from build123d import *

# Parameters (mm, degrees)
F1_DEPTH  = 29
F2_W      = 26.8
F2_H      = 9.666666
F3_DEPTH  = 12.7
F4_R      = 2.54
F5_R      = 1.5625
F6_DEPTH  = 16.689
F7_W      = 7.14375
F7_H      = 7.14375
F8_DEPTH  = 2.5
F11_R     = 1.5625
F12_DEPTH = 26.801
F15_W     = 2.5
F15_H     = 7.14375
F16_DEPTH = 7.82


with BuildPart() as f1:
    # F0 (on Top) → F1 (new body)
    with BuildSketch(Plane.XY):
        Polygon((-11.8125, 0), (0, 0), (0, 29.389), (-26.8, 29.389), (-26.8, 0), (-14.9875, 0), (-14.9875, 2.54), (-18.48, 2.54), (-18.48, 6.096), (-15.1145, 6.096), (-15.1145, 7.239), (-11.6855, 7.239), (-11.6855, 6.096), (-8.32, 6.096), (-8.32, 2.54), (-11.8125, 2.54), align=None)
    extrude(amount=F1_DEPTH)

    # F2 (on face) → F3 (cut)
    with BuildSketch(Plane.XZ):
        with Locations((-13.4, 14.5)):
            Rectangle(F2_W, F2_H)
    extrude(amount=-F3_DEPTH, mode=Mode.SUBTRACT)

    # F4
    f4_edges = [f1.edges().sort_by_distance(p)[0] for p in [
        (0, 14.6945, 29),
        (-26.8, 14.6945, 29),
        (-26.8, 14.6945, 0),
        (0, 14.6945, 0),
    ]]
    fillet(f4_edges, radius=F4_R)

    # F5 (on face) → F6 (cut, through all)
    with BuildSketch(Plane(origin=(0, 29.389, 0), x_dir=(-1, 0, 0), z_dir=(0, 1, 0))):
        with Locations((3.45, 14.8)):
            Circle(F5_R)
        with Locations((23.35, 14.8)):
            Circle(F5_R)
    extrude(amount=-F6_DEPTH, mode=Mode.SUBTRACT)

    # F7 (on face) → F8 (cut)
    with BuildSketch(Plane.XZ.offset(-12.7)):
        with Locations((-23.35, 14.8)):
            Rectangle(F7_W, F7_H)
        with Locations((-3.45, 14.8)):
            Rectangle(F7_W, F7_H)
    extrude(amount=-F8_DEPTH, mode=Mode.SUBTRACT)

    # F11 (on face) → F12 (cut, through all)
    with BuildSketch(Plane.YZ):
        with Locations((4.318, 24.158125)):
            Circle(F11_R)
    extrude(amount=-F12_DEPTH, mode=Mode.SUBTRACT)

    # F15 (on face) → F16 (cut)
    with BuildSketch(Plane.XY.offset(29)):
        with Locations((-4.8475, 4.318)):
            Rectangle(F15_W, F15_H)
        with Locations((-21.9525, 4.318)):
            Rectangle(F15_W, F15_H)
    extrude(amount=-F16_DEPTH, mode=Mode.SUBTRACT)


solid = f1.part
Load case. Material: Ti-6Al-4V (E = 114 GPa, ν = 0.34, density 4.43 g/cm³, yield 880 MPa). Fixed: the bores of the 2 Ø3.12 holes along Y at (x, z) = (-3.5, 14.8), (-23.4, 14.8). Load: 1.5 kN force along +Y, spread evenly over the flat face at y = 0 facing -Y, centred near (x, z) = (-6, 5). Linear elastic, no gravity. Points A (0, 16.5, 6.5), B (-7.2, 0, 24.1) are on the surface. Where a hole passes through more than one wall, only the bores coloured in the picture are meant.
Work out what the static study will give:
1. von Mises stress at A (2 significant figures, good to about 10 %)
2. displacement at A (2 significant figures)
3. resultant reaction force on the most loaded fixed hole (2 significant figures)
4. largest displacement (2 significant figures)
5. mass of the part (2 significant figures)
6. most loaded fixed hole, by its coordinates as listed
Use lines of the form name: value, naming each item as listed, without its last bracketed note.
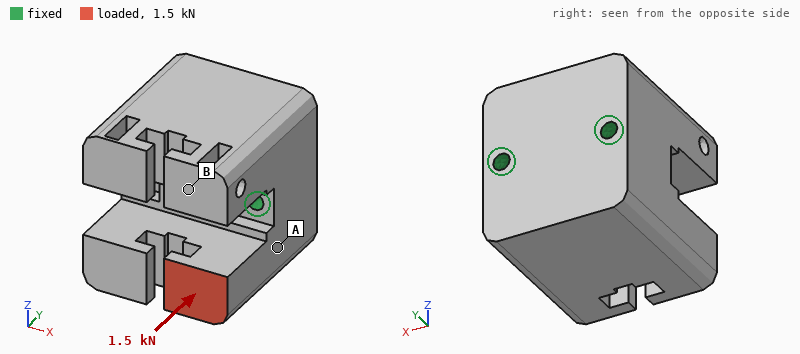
von Mises stress at A: 18 MPa
displacement at A: 3.1 µm
resultant reaction force on the most loaded fixed hole: 1.2 kN
largest displacement: 14 µm
mass of the part: 78 g
most loaded fixed hole, by its coordinates as listed: (-3.5, 14.8)
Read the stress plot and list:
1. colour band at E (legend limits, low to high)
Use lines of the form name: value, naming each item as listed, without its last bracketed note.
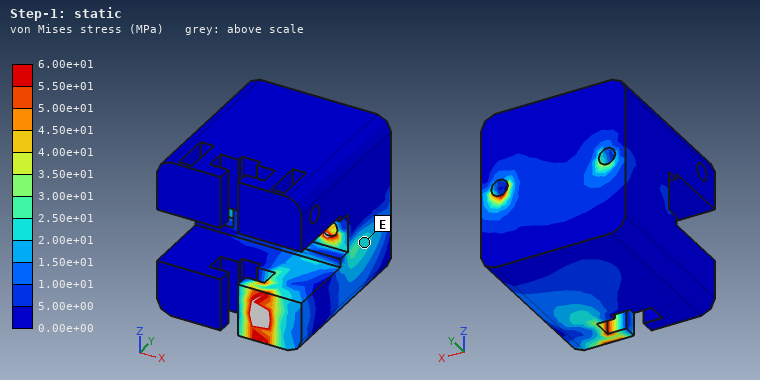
colour band at E: 2.00e+01 to 2.50e+01 MPa
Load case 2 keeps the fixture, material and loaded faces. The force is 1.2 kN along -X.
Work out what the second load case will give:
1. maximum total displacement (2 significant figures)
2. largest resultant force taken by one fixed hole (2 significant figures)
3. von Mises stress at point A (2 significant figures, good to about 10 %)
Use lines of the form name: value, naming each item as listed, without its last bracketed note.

maximum total displacement: 24 µm
largest resultant force taken by one fixed hole: 1.4 kN
von Mises stress at point A: 33 MPa
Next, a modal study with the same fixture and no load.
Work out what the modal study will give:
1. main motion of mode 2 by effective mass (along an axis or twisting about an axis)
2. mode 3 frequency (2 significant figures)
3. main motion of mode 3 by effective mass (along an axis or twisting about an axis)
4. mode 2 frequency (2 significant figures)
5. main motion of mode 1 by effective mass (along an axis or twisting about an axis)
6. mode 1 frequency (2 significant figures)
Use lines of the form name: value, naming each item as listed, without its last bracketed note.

main motion of mode 2 by effective mass: along Y
mode 3 frequency: 21 kHz
main motion of mode 3 by effective mass: along X
mode 2 frequency: 19 kHz
main motion of mode 1 by effective mass: along Z
mode 1 frequency: 14 kHz
